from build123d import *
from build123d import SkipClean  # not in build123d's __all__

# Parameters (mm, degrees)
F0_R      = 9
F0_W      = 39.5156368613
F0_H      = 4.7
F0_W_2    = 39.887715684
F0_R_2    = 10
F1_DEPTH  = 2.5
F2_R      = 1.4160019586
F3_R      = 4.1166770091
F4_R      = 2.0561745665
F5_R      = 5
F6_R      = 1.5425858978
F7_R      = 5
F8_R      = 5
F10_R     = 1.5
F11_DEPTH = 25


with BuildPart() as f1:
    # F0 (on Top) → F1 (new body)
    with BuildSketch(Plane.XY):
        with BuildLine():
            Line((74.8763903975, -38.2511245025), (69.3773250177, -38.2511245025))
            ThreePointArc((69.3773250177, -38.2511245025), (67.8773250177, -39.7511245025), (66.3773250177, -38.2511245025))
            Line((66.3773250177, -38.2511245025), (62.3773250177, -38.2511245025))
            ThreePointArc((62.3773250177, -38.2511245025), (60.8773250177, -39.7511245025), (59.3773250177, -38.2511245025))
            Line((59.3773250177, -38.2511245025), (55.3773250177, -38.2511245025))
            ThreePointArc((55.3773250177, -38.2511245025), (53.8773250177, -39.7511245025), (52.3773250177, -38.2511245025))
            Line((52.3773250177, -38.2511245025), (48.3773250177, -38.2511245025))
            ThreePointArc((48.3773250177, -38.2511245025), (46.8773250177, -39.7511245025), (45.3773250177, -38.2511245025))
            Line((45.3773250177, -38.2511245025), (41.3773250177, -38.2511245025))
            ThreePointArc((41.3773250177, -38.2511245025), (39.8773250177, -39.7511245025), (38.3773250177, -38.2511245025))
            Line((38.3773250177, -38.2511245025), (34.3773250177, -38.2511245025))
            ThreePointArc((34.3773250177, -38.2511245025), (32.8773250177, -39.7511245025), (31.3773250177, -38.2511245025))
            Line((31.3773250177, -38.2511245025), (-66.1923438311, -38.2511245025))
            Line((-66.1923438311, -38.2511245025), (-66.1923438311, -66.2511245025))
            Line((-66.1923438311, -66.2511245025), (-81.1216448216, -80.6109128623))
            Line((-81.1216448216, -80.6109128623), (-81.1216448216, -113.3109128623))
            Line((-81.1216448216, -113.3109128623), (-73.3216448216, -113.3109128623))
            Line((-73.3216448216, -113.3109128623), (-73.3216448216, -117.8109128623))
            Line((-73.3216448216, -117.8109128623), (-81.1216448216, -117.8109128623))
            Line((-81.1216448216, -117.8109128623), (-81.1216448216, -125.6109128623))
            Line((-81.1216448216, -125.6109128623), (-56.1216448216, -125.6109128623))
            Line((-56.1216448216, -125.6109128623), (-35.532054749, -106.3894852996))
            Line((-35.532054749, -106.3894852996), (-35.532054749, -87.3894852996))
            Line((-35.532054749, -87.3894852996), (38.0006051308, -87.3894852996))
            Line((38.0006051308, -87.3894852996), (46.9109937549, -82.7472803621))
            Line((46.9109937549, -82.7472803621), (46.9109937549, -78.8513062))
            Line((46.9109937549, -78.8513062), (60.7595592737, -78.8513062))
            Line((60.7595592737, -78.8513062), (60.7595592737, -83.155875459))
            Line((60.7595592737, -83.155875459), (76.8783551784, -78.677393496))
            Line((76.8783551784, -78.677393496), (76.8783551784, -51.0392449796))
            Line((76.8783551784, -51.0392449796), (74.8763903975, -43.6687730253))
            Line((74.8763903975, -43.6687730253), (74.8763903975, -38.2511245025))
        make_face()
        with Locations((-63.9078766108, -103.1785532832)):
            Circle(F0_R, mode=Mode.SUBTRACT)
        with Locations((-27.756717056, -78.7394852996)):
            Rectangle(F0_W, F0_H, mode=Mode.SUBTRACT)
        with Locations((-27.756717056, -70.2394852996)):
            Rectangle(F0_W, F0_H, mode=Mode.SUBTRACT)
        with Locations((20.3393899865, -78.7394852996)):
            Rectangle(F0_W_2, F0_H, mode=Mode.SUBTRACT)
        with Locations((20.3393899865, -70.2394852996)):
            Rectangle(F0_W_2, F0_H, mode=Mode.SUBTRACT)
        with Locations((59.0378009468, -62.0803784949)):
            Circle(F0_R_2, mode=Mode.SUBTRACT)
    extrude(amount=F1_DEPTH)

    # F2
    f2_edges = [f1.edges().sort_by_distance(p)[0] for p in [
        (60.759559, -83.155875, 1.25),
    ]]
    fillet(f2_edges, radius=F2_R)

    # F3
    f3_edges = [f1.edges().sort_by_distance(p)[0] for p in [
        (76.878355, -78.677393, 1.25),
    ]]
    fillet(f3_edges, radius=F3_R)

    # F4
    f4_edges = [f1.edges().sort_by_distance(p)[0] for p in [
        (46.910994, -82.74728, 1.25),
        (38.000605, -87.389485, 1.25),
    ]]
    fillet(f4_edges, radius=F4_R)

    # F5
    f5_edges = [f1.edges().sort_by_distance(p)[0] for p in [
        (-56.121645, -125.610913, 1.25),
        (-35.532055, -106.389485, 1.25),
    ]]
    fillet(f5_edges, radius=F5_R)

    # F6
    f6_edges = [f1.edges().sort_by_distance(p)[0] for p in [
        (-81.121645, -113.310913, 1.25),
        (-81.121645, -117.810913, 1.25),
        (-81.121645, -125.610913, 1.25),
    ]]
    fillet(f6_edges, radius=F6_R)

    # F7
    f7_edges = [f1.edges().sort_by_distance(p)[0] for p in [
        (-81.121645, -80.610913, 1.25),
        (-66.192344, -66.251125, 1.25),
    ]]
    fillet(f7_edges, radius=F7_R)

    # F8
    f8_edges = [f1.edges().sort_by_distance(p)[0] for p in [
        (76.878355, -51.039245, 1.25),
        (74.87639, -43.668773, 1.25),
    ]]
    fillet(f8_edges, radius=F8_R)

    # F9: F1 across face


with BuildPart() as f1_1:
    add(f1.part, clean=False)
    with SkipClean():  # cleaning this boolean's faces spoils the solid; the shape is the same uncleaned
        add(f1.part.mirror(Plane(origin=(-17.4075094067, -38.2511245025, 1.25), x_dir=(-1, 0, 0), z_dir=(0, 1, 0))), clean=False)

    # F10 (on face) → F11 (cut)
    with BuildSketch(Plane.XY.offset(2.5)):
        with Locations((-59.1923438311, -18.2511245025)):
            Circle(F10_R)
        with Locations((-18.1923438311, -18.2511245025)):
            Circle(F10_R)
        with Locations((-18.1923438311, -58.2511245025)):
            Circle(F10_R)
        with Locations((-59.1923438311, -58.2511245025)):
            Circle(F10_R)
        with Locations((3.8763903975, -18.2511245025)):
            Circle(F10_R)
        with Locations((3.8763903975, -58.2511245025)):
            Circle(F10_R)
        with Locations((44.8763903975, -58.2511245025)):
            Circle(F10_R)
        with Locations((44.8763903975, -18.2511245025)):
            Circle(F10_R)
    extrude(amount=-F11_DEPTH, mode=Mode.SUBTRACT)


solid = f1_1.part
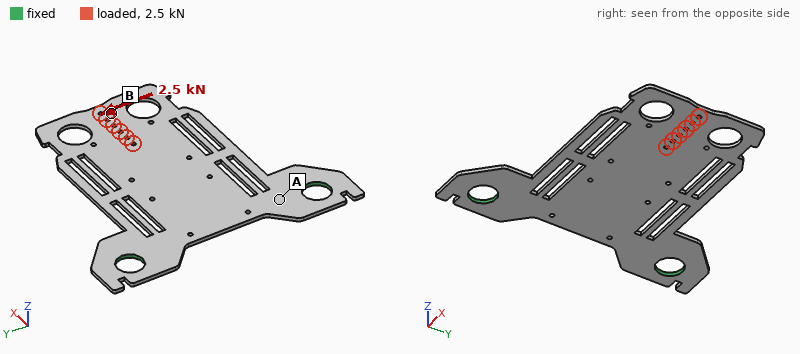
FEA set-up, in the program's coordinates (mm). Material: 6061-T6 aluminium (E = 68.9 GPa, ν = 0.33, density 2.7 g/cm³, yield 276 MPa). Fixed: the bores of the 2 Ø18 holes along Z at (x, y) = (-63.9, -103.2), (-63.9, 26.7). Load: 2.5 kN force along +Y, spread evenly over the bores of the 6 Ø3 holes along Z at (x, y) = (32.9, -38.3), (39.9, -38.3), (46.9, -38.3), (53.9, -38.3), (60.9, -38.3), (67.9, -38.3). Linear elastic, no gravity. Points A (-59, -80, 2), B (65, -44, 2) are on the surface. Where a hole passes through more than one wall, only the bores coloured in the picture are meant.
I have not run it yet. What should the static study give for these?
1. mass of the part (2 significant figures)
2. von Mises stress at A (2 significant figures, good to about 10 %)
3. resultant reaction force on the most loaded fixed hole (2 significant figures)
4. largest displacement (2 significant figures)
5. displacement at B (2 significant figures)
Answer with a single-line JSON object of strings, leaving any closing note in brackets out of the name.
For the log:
{"mass of the part": "96 g", "von Mises stress at A": "62 MPa", "resultant reaction force on the most loaded fixed hole": "3.2 kN", "largest displacement": "0.43 mm", "displacement at B": "0.39 mm"}
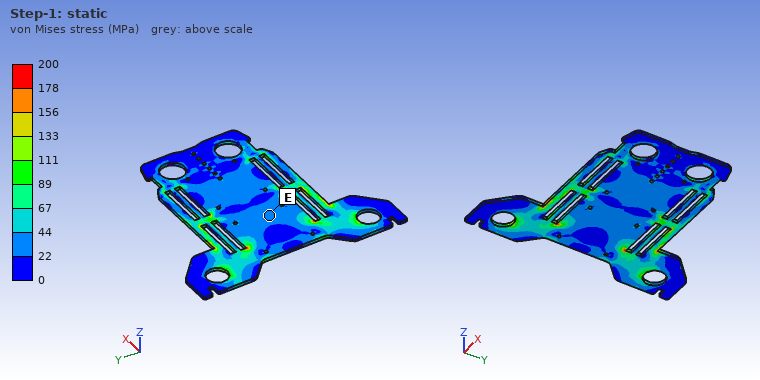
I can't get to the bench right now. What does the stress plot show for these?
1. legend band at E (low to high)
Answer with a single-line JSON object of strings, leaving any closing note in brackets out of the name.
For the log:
{"legend band at E": "22 to 44 MPa"}
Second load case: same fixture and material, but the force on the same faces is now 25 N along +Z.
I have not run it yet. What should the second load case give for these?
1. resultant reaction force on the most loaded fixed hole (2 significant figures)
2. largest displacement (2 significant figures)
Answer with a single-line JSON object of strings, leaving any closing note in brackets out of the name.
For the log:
{"resultant reaction force on the most loaded fixed hole": "13 N", "largest displacement": "2.5 mm"}
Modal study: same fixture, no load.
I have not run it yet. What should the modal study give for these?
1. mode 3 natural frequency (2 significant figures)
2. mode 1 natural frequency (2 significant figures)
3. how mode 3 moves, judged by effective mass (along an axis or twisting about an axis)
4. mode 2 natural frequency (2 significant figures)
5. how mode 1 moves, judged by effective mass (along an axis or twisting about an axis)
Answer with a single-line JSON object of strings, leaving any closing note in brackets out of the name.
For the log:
{"mode 3 natural frequency": "590 Hz", "mode 1 natural frequency": "110 Hz", "how mode 3 moves, judged by effective mass": "along Z", "mode 2 natural frequency": "410 Hz", "how mode 1 moves, judged by effective mass": "along Z"}
